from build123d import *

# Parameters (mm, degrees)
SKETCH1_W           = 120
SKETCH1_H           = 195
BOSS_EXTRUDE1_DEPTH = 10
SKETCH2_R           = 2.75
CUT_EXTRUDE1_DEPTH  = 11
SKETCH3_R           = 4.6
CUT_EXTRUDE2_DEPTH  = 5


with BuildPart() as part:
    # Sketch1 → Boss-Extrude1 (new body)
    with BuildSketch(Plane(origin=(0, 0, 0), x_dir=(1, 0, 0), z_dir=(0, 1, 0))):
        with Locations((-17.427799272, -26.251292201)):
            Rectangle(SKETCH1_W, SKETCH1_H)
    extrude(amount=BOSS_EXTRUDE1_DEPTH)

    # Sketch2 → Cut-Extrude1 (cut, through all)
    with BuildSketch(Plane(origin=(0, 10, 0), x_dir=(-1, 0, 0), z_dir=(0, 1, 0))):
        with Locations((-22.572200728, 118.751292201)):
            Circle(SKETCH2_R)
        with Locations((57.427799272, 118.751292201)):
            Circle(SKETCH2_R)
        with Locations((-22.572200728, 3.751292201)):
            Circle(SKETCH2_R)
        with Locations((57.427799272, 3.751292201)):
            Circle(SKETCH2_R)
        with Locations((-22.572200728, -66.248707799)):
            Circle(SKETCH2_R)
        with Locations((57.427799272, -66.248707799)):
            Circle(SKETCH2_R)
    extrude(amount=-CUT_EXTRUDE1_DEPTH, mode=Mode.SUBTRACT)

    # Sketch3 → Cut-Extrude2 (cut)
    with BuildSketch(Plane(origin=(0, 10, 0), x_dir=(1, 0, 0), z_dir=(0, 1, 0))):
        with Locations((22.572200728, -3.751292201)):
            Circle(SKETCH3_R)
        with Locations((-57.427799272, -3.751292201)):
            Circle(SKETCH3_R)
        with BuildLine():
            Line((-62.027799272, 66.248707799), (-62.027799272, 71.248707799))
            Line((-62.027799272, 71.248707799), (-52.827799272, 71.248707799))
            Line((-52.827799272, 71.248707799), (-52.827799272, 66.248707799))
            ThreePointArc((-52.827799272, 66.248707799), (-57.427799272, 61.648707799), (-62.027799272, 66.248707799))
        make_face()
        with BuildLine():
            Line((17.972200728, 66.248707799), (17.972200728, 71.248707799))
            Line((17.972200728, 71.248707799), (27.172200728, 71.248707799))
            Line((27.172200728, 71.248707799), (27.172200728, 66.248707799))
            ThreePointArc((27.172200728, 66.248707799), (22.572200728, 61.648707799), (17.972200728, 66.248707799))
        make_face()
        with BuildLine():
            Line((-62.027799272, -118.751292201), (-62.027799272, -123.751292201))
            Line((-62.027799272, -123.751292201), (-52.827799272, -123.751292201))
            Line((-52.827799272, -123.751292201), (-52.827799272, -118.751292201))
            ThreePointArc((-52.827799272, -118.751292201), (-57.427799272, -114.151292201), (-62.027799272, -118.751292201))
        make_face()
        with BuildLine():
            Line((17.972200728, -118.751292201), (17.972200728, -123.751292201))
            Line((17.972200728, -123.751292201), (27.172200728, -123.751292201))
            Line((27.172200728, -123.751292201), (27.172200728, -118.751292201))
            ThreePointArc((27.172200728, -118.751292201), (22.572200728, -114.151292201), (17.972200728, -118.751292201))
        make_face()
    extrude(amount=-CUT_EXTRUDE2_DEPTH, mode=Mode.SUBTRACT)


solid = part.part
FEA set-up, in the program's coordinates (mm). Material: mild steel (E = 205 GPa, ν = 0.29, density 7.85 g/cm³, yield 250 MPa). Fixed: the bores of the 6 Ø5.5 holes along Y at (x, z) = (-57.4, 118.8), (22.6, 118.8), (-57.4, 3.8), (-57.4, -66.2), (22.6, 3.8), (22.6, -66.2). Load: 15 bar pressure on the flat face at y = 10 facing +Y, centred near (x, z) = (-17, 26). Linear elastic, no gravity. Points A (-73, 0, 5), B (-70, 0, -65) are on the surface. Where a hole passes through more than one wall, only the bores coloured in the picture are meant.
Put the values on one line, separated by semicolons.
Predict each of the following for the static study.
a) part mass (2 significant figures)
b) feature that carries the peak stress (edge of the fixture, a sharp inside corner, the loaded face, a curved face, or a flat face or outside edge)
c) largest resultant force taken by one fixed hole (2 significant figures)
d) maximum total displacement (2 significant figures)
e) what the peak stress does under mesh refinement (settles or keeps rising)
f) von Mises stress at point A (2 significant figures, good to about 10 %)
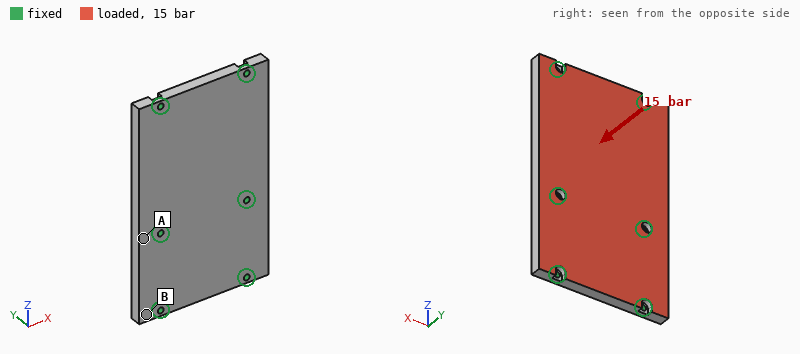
1.8 kg; edge of the fixture; 11 kN; 93 µm; keeps rising; 82 MPa
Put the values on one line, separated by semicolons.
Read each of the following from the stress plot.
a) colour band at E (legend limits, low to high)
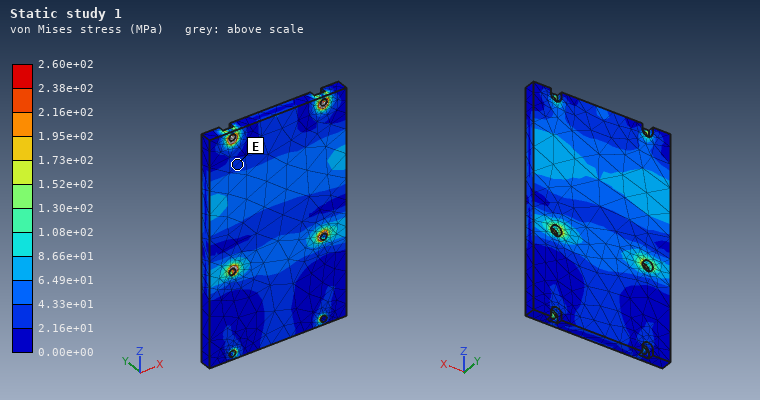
2.16e+01 to 4.33e+01 MPa
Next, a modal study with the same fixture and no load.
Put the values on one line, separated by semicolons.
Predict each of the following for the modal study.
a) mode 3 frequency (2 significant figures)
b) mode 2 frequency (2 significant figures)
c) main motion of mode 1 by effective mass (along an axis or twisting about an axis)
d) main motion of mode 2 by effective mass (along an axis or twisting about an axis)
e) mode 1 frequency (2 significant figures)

4400 Hz; 3500 Hz; along Y; twisting about Z; 2600 Hz
